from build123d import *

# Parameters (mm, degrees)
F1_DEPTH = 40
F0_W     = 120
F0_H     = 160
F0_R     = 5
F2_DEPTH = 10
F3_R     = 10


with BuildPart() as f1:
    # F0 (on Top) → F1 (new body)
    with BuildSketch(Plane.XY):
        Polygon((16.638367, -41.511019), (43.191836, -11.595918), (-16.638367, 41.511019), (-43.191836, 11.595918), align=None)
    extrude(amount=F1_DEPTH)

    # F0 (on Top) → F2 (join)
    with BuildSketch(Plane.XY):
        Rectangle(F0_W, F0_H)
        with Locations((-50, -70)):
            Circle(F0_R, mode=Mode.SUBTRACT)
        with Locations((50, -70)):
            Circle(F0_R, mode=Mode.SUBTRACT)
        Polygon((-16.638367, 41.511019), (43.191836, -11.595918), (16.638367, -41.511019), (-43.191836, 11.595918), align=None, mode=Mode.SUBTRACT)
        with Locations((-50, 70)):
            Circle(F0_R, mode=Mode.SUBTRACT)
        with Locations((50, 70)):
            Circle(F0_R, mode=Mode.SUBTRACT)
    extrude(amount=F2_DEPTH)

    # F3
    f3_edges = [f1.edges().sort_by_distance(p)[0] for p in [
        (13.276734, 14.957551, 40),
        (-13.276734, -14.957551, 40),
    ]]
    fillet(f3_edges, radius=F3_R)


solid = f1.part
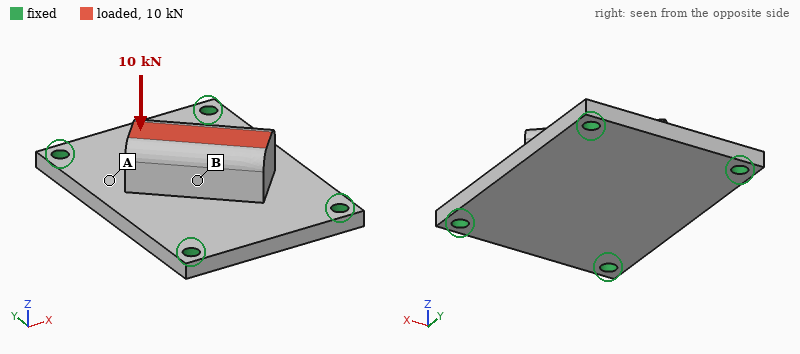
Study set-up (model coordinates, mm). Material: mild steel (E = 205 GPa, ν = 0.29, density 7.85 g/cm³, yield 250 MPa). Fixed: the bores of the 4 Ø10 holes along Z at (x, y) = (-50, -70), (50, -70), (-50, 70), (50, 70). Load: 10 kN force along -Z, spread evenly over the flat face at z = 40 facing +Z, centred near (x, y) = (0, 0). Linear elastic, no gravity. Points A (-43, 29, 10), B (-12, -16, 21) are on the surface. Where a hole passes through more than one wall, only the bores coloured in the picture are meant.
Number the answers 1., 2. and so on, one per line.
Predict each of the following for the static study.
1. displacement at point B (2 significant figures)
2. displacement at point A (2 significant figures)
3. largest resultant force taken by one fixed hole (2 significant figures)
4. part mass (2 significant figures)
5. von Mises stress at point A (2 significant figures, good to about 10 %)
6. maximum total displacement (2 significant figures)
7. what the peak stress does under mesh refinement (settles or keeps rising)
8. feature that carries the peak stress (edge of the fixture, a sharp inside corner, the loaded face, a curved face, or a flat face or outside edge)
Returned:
1. 48 µm
2. 39 µm
3. 3.5 kN
4. 2.2 kg
5. 38 MPa
6. 48 µm
7. keeps rising
8. edge of the fixture
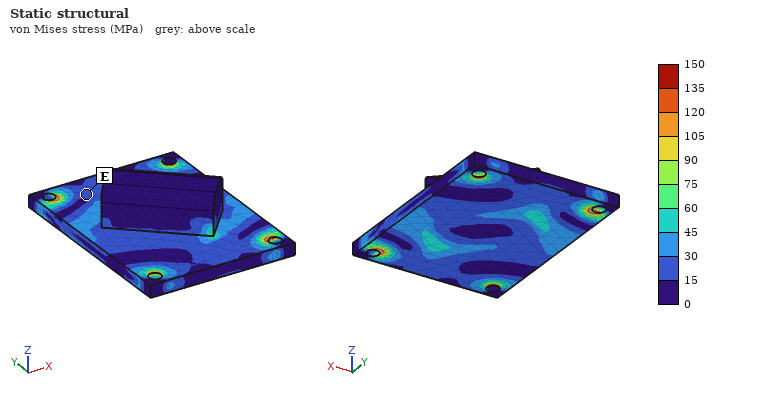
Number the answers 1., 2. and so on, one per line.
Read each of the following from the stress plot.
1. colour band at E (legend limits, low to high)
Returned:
1. 15 to 30 MPa
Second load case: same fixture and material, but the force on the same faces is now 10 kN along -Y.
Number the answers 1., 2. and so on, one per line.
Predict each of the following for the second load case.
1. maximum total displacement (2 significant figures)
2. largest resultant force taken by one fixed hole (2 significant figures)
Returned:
1. 33 µm
2. 3.3 kN
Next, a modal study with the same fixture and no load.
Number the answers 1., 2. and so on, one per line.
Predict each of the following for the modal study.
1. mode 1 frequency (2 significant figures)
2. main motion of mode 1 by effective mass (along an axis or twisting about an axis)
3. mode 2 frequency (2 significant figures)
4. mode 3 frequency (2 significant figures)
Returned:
1. 1900 Hz
2. along Z
3. 2600 Hz
4. 3800 Hz
